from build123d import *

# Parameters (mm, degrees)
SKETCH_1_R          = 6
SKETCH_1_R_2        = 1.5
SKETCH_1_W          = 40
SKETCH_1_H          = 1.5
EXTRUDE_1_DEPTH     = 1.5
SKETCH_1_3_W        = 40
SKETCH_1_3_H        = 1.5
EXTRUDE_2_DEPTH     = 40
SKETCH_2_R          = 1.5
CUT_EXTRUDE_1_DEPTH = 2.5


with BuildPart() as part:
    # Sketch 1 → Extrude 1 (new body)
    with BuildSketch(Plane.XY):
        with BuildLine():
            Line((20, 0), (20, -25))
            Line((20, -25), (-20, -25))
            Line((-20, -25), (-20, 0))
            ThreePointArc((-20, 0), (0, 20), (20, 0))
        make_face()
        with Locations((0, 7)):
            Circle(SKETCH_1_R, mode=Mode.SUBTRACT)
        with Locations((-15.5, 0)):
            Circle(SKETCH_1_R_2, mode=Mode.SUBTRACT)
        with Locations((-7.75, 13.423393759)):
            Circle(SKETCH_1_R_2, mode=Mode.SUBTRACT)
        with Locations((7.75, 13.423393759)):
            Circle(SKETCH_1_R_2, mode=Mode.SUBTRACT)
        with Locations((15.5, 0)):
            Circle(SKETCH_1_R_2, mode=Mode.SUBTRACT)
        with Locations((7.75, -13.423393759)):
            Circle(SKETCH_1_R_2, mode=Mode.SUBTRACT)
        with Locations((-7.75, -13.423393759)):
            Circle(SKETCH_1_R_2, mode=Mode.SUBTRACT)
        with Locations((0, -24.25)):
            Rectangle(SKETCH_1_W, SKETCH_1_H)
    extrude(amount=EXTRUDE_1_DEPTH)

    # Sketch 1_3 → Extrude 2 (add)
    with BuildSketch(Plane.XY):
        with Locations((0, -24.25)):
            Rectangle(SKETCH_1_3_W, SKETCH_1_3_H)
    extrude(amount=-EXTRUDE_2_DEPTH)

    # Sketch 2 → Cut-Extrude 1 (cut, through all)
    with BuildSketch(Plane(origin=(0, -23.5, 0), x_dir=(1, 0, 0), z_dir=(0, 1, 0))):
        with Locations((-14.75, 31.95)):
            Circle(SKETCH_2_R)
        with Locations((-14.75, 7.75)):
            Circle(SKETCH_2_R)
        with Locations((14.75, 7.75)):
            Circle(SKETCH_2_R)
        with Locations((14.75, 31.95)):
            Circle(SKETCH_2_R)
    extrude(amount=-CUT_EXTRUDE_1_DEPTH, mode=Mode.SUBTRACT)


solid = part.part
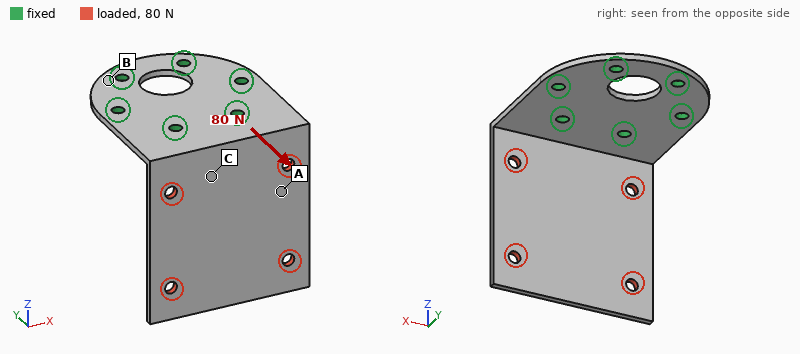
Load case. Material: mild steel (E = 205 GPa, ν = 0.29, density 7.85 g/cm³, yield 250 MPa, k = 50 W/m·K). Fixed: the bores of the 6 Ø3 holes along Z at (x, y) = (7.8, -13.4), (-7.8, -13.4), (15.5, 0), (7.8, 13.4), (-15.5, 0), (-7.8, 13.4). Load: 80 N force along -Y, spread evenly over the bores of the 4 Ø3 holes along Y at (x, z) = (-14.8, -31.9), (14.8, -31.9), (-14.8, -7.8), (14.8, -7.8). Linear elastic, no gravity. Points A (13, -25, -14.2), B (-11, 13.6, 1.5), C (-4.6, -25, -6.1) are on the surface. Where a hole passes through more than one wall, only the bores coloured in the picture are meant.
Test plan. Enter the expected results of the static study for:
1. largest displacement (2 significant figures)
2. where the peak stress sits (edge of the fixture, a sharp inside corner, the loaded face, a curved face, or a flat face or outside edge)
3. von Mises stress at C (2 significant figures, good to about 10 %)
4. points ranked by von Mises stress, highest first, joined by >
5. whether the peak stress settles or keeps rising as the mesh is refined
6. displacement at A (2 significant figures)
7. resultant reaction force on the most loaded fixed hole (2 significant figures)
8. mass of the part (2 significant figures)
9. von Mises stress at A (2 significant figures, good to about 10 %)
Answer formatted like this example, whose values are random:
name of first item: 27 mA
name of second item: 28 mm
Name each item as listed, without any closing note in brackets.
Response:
largest displacement: 0.57 mm
where the peak stress sits: edge of the fixture
von Mises stress at C: 71 MPa
points ranked by von Mises stress, highest first, joined by >: C > A > B
whether the peak stress settles or keeps rising as the mesh is refined: keeps rising
displacement at A: 0.17 mm
resultant reaction force on the most loaded fixed hole: 37 N
mass of the part: 36 g
von Mises stress at A: 43 MPa
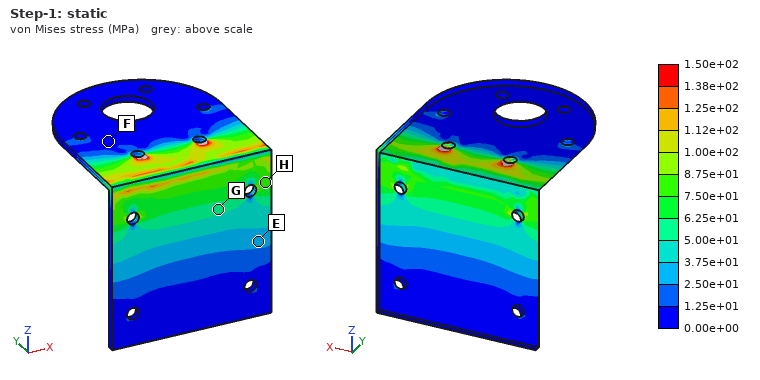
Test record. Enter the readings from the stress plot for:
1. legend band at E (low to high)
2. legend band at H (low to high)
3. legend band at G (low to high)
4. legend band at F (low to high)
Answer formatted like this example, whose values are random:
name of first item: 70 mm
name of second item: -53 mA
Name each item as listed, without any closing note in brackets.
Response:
legend band at E: 2.50e+01 to 3.75e+01 MPa
legend band at H: 7.50e+01 to 8.75e+01 MPa
legend band at G: 5.00e+01 to 6.25e+01 MPa
legend band at F: 0.00e+00 to 1.25e+01 MPa
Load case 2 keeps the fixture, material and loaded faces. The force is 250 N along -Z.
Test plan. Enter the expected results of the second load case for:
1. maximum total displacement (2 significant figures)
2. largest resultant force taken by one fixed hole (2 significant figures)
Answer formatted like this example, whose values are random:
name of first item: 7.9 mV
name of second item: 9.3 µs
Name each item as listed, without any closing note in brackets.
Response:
maximum total displacement: 0.26 mm
largest resultant force taken by one fixed hole: 150 N
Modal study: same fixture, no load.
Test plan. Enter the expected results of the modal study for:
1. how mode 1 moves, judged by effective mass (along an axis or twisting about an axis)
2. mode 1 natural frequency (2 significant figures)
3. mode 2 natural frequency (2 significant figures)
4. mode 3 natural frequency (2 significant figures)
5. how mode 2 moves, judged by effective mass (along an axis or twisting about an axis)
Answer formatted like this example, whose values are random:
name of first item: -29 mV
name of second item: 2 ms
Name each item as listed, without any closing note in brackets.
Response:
how mode 1 moves, judged by effective mass: along Y
mode 1 natural frequency: 540 Hz
mode 2 natural frequency: 1300 Hz
mode 3 natural frequency: 1900 Hz
how mode 2 moves, judged by effective mass: along X
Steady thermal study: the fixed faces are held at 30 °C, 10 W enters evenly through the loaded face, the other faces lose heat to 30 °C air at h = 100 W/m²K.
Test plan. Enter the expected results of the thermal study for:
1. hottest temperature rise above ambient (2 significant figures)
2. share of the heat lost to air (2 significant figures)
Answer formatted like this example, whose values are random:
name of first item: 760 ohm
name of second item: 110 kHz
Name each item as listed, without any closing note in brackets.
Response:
hottest temperature rise above ambient: 35 K
share of the heat lost to air: 77 %
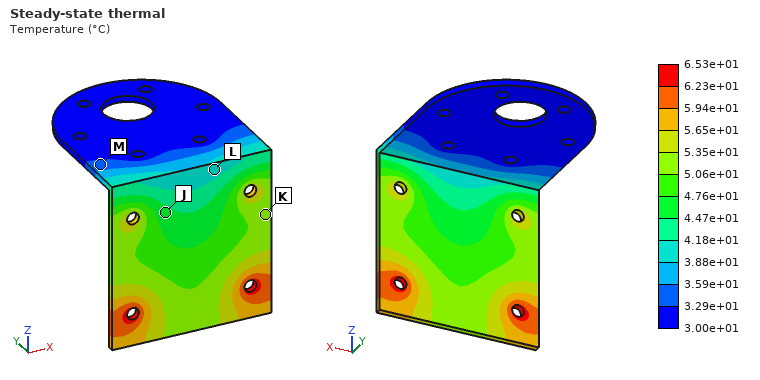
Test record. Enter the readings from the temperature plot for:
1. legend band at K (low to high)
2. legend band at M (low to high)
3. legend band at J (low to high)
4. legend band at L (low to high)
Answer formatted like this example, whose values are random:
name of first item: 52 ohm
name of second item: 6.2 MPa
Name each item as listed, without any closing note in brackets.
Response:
legend band at K: 5.06e+01 to 5.35e+01 °C
legend band at M: 3.29e+01 to 3.59e+01 °C
legend band at J: 4.47e+01 to 4.76e+01 °C
legend band at L: 3.88e+01 to 4.18e+01 °C
